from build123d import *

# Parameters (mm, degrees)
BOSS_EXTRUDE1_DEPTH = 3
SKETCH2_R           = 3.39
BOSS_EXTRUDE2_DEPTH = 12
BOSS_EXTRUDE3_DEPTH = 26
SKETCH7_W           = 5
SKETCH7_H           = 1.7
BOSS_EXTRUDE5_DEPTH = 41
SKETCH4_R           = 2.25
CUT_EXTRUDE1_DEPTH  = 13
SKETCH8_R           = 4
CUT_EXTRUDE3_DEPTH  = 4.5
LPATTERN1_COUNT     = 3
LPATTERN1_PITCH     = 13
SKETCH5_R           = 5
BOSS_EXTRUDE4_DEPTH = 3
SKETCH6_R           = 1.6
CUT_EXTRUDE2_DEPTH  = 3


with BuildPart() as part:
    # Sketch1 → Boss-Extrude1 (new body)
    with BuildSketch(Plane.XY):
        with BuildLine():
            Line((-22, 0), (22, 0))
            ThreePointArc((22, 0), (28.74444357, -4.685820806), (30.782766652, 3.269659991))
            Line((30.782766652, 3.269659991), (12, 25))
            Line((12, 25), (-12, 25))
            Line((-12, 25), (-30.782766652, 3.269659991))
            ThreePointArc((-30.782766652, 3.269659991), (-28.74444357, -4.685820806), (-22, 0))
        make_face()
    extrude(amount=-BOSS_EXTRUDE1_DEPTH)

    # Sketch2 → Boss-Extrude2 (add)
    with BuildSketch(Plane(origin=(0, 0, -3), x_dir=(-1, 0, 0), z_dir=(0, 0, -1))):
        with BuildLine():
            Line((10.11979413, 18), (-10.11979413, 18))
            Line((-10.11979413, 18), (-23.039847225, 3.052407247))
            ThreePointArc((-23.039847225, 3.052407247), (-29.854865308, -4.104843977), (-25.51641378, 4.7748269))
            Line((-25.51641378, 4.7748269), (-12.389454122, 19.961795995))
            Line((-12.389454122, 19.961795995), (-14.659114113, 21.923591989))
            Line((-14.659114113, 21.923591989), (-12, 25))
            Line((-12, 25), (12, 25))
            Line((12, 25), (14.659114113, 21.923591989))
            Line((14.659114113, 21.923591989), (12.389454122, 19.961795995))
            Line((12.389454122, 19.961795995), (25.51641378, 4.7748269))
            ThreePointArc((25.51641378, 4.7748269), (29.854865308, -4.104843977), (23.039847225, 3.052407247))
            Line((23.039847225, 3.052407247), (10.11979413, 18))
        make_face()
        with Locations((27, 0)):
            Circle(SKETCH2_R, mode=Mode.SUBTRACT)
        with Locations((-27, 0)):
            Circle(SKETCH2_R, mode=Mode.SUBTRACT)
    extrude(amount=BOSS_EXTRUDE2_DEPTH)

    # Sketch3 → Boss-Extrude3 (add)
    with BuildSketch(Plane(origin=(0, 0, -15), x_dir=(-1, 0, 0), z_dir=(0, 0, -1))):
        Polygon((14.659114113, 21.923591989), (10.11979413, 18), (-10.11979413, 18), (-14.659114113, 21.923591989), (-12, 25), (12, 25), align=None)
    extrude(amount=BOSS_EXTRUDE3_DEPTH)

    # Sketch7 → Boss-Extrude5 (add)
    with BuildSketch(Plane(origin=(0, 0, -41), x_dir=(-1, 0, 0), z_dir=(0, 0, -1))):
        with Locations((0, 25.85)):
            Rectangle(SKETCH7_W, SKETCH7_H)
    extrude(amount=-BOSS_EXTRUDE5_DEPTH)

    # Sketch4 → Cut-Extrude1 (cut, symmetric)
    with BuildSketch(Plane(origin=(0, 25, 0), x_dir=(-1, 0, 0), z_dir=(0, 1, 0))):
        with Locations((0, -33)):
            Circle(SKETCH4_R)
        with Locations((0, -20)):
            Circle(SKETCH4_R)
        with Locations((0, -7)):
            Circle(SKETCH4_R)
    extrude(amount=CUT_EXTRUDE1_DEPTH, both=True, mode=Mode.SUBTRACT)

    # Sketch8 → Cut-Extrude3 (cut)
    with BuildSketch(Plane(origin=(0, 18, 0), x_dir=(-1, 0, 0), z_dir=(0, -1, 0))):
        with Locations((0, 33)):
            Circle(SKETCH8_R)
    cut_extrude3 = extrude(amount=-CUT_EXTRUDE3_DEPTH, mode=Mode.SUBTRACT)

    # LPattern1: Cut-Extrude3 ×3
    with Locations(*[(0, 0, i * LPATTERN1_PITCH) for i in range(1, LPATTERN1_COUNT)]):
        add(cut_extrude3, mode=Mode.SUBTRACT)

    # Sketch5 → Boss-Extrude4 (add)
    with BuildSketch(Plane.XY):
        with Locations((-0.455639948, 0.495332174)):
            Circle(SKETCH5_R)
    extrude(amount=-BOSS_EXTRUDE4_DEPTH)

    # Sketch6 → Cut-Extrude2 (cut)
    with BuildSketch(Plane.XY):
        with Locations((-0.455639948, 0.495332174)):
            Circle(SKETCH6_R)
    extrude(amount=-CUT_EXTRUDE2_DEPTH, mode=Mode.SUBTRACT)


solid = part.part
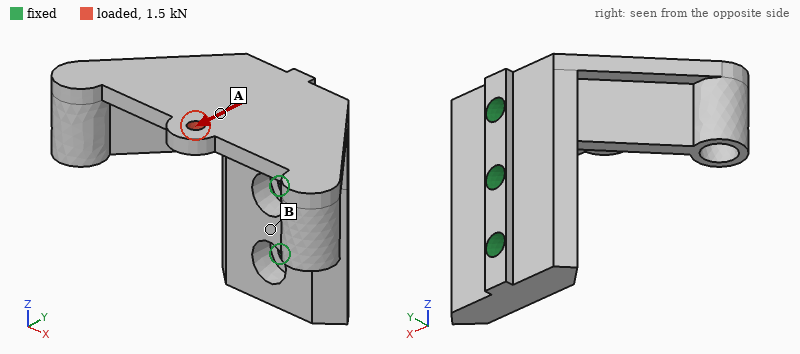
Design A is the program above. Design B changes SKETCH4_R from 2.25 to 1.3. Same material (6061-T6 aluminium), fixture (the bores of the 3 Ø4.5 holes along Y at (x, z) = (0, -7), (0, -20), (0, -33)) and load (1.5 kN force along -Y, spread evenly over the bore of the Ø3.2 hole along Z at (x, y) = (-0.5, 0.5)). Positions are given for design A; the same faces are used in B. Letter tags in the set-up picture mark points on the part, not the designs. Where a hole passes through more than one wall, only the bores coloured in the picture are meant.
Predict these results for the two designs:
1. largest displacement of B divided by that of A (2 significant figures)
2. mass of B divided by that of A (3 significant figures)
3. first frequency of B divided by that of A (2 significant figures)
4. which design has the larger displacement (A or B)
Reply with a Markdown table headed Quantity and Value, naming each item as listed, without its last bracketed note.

| Quantity | Value |
|---|---|
| largest displacement of B divided by that of A | 1.3 |
| mass of B divided by that of A | 1.01 |
| first frequency of B divided by that of A | 0.85 |
| which design has the larger displacement | B |
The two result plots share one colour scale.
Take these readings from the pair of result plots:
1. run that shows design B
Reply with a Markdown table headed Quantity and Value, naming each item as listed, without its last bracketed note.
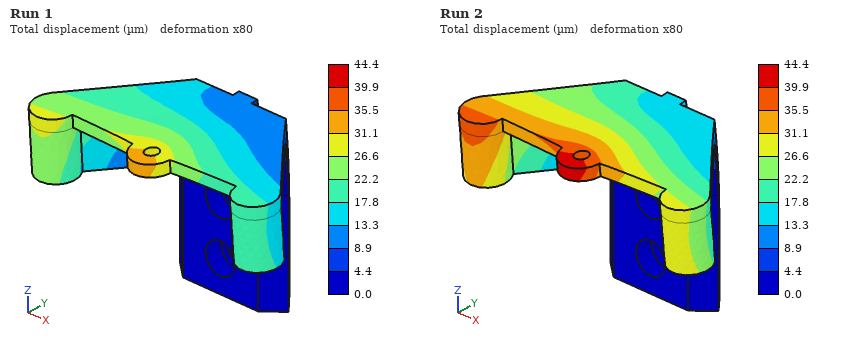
| Quantity | Value |
|---|---|
| run that shows design B | Run 2 |
